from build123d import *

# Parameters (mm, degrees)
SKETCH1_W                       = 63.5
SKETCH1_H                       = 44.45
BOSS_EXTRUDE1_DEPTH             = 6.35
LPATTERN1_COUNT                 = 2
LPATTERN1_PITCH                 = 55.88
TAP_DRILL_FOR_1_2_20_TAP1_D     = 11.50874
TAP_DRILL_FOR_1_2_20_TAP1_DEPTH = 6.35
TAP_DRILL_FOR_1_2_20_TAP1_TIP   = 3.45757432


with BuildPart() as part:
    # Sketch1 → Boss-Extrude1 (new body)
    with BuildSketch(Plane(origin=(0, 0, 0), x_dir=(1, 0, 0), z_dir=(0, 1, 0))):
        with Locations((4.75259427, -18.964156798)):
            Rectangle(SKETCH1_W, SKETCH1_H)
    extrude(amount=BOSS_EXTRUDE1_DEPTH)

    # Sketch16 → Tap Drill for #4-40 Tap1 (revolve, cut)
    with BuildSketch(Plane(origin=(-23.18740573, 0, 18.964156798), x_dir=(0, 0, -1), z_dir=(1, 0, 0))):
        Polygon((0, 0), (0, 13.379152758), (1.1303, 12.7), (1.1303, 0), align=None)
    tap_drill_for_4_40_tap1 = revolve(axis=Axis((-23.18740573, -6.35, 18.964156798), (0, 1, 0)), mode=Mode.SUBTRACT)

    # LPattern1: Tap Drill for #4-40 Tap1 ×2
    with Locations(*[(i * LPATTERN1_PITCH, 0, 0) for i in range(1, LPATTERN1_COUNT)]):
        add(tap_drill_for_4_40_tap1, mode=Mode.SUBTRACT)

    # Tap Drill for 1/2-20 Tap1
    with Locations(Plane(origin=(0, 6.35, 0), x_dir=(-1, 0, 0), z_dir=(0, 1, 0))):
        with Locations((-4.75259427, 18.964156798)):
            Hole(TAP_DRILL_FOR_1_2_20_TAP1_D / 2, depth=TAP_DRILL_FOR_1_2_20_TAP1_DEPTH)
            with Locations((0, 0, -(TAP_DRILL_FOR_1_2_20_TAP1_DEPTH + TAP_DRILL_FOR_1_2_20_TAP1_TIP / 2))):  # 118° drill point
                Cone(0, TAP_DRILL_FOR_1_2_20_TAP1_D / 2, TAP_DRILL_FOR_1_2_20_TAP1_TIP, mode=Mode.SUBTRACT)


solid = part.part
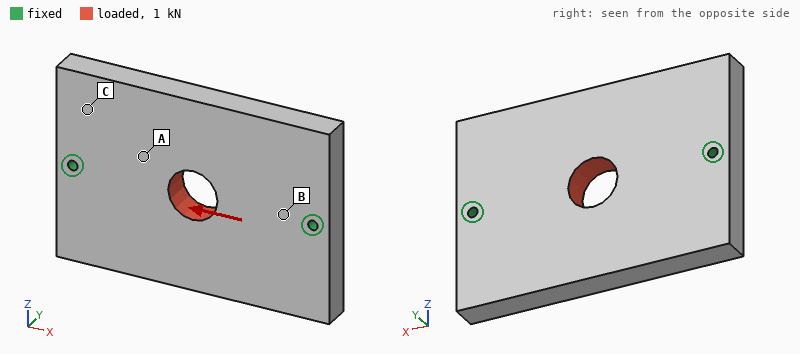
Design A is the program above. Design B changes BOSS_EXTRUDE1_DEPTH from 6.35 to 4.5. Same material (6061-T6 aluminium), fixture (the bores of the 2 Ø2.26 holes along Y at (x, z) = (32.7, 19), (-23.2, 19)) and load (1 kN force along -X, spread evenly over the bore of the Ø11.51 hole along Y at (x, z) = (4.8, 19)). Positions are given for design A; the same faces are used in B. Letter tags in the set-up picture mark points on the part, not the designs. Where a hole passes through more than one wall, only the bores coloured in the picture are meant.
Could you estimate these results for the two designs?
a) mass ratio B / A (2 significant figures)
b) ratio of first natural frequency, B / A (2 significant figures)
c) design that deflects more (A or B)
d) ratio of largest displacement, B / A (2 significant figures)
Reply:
0.71
0.75
B
1.4
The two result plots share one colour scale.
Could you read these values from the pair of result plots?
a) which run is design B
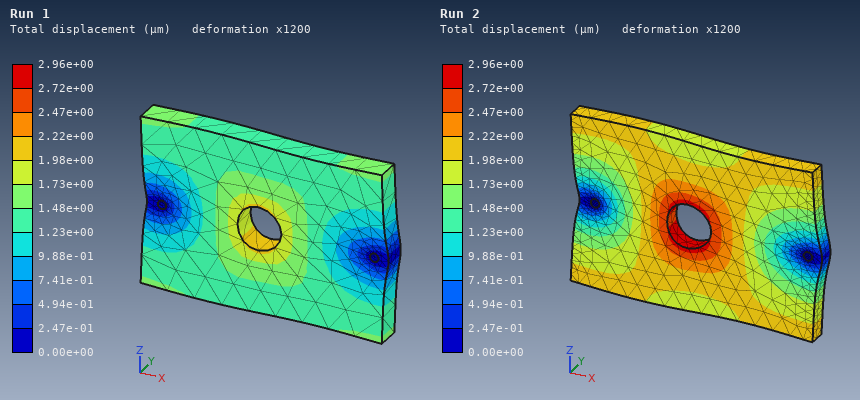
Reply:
Run 2
